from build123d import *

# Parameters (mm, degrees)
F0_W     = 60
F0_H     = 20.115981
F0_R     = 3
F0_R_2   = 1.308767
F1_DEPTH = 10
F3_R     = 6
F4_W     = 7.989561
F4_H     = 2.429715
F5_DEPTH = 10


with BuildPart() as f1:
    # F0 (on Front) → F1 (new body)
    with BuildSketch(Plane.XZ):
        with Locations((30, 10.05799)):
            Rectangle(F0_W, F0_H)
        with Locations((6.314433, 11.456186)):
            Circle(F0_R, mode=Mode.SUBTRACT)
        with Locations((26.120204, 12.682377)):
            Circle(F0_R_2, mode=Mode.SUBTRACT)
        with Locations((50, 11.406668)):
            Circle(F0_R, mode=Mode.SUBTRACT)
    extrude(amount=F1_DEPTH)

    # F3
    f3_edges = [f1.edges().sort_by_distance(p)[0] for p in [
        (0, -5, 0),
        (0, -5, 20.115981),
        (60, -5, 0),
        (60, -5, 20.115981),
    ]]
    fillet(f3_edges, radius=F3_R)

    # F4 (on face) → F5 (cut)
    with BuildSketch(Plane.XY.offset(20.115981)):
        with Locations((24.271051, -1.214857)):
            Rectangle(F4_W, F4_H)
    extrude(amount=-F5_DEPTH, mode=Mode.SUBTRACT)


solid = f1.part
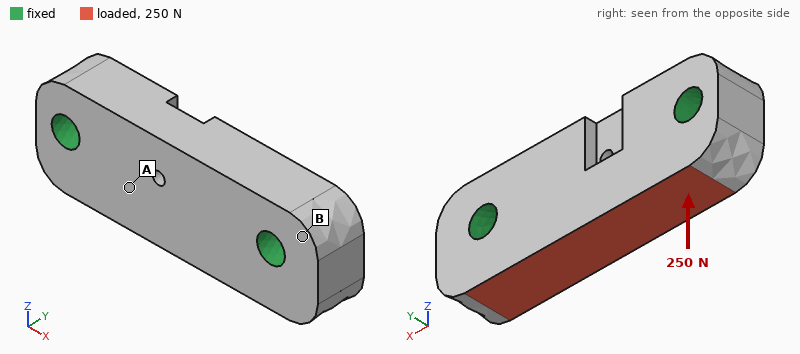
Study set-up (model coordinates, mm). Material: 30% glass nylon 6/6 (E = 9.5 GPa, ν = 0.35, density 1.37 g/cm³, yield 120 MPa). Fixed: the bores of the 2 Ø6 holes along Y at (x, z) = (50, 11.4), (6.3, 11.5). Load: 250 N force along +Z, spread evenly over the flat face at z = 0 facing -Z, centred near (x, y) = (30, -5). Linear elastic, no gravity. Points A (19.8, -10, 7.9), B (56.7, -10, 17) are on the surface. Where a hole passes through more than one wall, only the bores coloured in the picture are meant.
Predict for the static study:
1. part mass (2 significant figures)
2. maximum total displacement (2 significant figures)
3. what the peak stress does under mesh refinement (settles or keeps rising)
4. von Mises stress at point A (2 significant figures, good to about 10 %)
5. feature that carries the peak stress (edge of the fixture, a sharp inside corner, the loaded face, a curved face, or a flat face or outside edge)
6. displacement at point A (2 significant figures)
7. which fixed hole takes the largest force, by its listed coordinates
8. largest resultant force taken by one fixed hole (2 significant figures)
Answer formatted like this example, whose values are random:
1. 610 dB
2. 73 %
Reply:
1. 15 g
2. 3.7 µm
3. keeps rising
4. 0.65 MPa
5. edge of the fixture
6. 2.8 µm
7. (50, 11.4)
8. 140 N
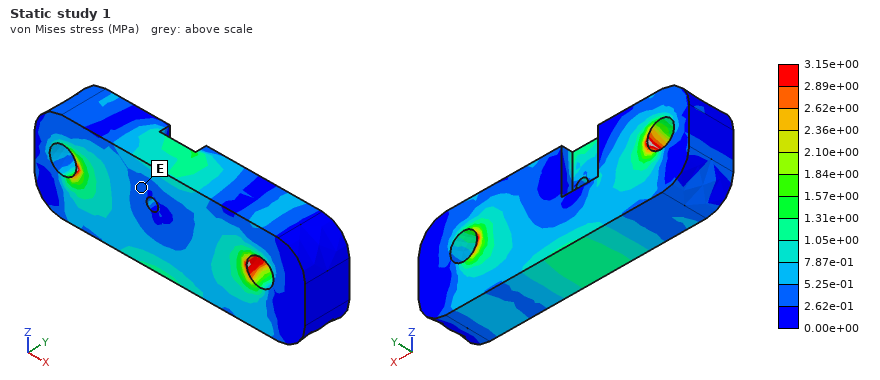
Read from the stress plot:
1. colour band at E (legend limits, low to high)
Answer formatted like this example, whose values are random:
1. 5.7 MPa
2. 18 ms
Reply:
1. 2.62e-01 to 5.25e-01 MPa
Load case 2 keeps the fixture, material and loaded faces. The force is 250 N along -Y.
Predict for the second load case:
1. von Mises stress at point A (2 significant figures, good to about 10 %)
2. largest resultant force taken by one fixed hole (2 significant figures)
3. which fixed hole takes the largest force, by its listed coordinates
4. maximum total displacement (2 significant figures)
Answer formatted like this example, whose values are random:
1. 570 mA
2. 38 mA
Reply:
1. 1.9 MPa
2. 140 N
3. (50, 11.4)
4. 16 µm
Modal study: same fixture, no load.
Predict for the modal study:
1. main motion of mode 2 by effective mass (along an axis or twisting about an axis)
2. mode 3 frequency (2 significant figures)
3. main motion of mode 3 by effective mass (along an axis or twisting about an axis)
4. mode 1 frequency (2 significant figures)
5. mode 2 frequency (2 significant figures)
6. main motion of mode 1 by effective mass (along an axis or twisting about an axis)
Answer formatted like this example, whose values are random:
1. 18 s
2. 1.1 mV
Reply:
1. along Z
2. 14 kHz
3. twisting about X
4. 11 kHz
5. 13 kHz
6. along Y
